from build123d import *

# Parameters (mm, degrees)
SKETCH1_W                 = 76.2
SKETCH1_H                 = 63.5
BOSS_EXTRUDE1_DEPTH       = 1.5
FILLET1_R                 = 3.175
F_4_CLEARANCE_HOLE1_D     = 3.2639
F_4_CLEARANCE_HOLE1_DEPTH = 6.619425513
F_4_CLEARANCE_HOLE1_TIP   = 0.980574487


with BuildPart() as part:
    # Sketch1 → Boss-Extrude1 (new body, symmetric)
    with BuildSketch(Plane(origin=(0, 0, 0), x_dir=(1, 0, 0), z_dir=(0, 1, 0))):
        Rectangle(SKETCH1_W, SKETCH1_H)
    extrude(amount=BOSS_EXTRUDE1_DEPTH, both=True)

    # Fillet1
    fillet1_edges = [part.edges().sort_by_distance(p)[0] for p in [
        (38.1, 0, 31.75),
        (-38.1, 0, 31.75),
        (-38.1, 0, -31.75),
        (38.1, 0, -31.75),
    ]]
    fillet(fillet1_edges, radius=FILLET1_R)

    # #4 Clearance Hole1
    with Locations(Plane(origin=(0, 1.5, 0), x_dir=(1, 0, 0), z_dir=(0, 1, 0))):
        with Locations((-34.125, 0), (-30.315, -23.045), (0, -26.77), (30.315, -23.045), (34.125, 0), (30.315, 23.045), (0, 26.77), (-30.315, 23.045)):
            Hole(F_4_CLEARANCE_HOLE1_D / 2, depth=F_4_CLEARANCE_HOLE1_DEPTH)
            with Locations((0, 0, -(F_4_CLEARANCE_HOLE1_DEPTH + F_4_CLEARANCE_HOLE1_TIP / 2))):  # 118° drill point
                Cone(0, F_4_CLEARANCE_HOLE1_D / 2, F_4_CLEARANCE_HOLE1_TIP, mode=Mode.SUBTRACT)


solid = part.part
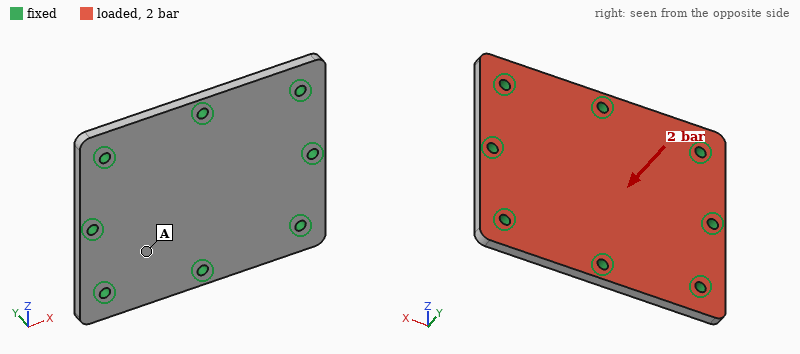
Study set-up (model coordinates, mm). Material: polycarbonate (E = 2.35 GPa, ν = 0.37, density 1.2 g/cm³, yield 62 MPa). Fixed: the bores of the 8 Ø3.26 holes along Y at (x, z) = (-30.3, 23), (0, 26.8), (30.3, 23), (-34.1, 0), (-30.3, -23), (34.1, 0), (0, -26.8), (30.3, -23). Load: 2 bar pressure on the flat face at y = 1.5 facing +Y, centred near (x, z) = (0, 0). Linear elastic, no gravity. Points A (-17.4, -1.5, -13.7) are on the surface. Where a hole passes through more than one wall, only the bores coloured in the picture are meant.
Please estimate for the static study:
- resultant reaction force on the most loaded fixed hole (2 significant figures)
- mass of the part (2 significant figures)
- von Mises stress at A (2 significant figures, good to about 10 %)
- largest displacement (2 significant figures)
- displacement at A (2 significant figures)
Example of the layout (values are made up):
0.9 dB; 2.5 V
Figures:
170 N; 17 g; 6.8 MPa; 0.65 mm; 0.30 mm
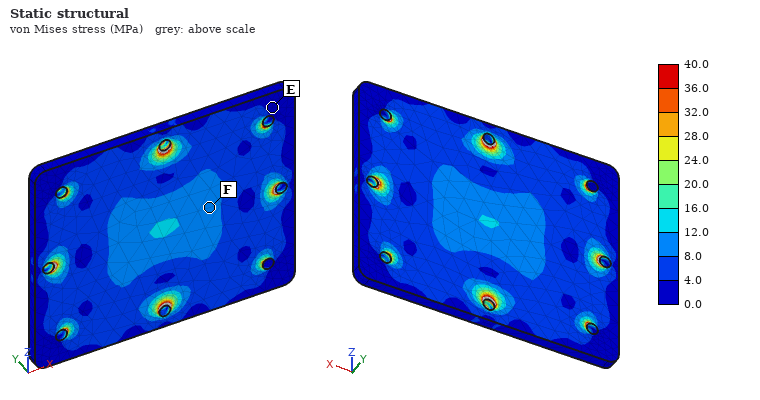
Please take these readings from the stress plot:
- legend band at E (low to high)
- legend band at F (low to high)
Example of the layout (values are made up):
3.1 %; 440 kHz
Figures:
0.0 to 4.0 MPa; 8.0 to 12.0 MPa
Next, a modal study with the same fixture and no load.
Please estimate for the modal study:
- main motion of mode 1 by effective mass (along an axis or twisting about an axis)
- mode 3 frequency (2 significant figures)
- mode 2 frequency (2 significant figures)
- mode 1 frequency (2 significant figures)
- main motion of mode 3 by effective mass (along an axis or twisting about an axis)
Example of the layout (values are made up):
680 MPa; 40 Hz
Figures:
along Y; 3800 Hz; 3000 Hz; 1800 Hz; twisting about X
